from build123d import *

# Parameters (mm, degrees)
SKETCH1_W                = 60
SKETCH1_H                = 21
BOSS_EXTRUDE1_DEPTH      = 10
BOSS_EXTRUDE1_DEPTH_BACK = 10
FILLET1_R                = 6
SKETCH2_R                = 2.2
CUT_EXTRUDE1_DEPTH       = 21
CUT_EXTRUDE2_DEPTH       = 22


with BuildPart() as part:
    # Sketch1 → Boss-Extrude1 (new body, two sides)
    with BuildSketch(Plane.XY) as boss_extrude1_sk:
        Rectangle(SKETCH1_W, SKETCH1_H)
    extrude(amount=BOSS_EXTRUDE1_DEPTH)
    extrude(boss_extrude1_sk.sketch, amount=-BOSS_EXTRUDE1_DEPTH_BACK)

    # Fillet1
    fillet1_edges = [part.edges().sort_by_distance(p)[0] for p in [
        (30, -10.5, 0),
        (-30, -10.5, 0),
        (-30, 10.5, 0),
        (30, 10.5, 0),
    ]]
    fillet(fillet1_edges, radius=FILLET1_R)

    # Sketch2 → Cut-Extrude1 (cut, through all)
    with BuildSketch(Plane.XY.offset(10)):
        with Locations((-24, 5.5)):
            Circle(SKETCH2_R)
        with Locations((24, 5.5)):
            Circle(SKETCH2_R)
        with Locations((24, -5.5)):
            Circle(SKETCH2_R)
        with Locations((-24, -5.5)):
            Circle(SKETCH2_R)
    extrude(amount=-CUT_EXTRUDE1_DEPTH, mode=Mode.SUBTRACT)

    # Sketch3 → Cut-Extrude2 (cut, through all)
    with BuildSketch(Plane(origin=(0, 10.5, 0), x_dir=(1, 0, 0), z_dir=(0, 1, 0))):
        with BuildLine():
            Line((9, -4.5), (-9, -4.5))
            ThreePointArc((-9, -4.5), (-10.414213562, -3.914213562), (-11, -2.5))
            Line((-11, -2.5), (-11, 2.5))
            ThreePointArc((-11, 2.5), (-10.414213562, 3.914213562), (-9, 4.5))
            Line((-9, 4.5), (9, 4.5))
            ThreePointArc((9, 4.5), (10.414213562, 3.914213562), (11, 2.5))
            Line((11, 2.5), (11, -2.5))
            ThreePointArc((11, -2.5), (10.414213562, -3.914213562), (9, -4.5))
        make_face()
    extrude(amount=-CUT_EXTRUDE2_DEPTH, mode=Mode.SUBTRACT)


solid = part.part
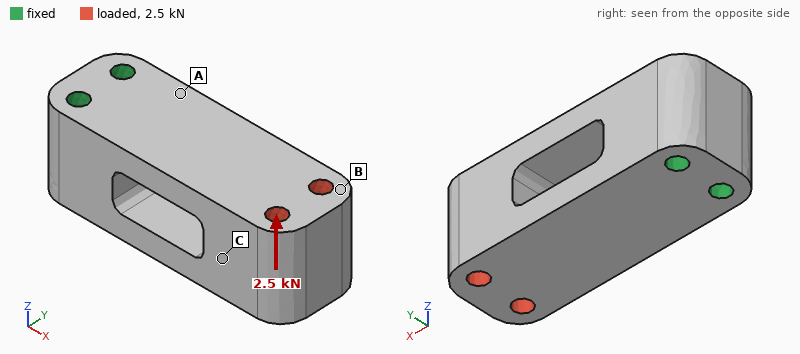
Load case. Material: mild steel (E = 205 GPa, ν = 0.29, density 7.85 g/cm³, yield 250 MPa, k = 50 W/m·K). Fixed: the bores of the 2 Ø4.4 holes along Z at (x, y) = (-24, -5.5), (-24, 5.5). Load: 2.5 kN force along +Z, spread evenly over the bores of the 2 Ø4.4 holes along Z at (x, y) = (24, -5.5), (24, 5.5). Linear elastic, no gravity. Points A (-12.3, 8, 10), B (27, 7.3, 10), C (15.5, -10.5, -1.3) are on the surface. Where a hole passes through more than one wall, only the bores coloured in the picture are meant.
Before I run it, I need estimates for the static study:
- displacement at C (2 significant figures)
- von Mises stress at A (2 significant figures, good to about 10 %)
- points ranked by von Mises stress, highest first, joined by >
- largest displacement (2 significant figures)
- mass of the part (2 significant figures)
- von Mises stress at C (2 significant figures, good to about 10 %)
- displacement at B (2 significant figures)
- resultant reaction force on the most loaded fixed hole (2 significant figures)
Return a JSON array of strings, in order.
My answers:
["56 µm", "120 MPa", "A > C > B", "72 µm", "150 g", "43 MPa", "69 µm", "1.3 kN"]
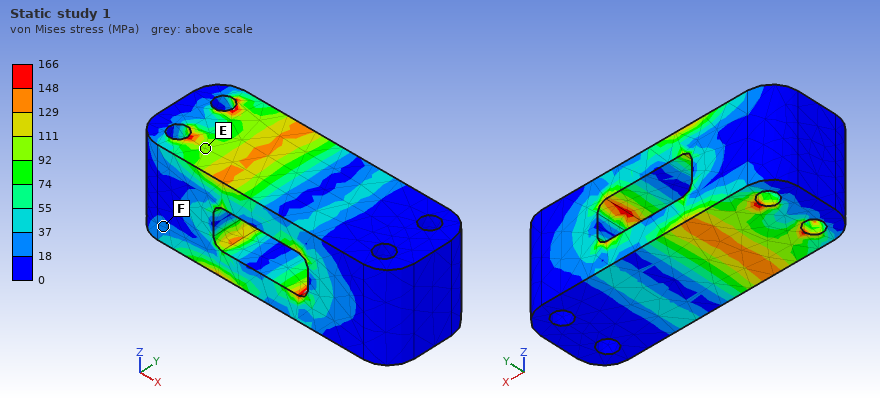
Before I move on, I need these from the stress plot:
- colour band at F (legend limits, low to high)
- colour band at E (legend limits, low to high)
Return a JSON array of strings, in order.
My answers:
["18 to 37 MPa", "92 to 111 MPa"]
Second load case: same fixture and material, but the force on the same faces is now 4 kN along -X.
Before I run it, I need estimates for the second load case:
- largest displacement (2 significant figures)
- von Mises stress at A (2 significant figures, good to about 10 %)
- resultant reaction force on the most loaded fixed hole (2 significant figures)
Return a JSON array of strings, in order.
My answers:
["3.7 µm", "18 MPa", "2.0 kN"]
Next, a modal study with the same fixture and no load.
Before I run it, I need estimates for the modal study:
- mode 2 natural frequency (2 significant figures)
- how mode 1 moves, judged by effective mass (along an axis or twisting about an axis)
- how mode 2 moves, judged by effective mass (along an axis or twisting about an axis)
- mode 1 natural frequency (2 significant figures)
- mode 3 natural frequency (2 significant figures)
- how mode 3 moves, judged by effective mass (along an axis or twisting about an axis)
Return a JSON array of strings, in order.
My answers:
["5100 Hz", "along Z", "along Y", "4100 Hz", "10 kHz", "twisting about X"]
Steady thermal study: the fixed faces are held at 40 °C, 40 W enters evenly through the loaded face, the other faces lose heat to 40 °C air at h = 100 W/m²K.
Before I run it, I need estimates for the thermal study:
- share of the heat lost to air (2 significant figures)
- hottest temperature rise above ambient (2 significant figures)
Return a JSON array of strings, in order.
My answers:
["53 %", "79 K"]
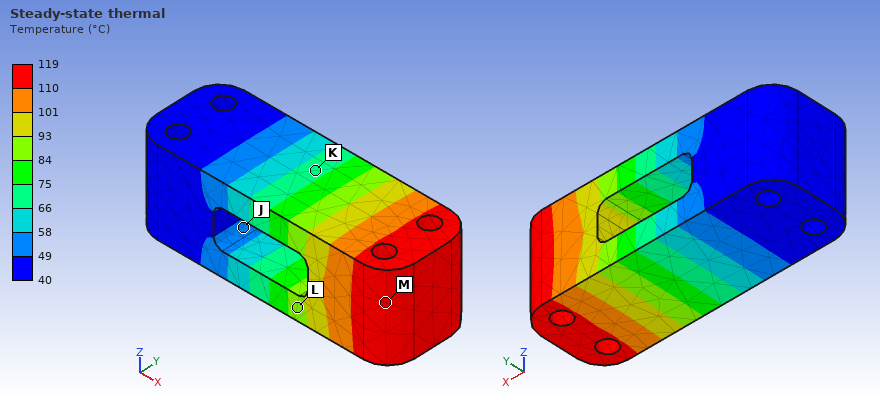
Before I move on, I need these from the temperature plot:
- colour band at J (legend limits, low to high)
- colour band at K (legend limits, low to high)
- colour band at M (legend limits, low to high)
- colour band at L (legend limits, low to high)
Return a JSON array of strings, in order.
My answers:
["49 to 58 °C", "66 to 75 °C", "110 to 119 °C", "84 to 93 °C"]
